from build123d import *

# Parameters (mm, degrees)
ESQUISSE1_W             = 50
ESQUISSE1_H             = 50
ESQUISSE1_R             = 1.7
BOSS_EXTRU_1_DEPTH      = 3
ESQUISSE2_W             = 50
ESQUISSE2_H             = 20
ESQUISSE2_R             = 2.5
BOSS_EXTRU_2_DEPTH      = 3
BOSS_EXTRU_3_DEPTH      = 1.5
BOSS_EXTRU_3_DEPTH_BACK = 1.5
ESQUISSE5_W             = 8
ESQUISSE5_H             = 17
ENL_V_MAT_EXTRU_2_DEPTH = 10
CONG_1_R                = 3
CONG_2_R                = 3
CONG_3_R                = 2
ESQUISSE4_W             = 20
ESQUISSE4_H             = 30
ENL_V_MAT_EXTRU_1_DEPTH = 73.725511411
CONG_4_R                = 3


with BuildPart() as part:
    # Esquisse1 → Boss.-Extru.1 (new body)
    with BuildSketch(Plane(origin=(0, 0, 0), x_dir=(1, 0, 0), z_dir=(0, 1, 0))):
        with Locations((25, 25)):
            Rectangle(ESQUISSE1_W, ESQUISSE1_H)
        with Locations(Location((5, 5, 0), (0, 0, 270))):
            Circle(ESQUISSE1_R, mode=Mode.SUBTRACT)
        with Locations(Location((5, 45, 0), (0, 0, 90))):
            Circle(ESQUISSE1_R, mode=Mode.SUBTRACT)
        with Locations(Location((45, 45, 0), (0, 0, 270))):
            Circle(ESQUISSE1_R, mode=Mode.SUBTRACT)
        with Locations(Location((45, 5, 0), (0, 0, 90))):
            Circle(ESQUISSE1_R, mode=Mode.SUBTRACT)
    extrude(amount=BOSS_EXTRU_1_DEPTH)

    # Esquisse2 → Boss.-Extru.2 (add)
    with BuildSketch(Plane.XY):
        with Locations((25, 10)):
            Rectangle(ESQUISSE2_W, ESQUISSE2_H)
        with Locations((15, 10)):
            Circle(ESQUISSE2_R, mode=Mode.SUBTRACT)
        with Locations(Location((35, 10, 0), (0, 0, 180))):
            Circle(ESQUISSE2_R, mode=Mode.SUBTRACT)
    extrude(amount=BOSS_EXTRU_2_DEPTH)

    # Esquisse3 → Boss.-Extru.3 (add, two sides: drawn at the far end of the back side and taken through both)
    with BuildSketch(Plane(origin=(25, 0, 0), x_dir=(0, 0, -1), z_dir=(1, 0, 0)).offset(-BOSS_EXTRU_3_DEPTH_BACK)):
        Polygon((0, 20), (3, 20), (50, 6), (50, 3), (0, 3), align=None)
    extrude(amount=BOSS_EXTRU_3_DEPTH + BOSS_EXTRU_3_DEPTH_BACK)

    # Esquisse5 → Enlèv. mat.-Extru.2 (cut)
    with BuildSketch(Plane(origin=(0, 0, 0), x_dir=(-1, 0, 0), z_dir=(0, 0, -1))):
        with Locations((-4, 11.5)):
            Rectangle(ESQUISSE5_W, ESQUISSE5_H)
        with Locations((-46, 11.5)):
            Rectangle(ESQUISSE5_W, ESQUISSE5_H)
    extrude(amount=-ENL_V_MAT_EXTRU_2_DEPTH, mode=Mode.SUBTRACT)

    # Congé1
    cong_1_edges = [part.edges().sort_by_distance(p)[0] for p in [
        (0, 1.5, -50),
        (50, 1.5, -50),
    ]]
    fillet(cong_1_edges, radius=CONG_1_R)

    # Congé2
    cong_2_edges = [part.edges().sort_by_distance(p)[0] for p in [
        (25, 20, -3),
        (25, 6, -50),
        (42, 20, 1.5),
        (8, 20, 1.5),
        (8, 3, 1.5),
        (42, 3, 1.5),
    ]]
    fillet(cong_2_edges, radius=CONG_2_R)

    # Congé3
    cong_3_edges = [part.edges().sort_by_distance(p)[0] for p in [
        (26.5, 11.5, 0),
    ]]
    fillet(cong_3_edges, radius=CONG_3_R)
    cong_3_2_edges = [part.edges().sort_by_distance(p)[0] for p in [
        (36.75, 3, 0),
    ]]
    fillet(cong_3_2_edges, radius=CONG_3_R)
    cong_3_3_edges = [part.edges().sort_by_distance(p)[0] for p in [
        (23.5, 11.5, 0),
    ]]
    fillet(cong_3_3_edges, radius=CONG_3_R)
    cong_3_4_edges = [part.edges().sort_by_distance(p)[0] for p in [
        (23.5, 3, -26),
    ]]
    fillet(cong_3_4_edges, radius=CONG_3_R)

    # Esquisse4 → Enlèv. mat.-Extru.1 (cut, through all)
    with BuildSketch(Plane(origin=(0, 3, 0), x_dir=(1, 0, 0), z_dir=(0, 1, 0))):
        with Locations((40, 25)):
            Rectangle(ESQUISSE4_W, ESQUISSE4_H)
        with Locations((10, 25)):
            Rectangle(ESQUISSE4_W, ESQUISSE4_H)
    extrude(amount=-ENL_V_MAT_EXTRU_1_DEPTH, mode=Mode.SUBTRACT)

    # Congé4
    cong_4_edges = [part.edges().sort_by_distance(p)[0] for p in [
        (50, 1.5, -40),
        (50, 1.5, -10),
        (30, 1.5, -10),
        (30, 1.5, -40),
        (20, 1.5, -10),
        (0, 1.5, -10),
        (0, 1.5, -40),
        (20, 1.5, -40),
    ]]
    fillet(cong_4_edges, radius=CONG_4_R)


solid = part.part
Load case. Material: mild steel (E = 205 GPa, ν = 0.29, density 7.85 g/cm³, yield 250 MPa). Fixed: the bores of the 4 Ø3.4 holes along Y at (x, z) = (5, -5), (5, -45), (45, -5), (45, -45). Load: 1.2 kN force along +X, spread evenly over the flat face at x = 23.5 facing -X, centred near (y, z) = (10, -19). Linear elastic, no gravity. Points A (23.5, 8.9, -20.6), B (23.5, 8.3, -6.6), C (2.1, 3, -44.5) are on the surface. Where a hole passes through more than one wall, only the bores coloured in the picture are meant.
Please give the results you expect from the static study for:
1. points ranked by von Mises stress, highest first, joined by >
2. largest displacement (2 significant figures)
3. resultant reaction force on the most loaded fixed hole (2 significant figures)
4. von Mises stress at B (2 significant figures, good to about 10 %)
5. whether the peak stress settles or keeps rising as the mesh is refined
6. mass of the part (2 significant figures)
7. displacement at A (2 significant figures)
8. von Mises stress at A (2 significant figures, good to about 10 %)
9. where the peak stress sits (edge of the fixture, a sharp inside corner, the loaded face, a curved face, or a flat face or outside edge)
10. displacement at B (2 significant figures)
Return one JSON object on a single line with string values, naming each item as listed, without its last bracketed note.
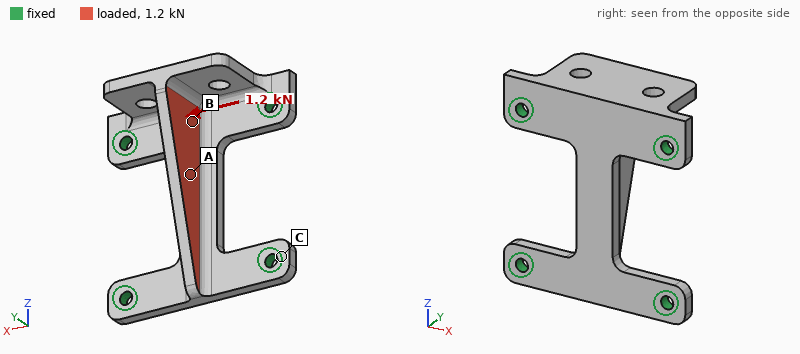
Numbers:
{"points ranked by von Mises stress, highest first, joined by >": "B > A > C", "largest displacement": "36 µm", "resultant reaction force on the most loaded fixed hole": "470 N", "von Mises stress at B": "58 MPa", "whether the peak stress settles or keeps rising as the mesh is refined": "keeps rising", "mass of the part": "59 g", "displacement at A": "21 µm", "von Mises stress at A": "33 MPa", "where the peak stress sits": "edge of the fixture", "displacement at B": "8.1 µm"}
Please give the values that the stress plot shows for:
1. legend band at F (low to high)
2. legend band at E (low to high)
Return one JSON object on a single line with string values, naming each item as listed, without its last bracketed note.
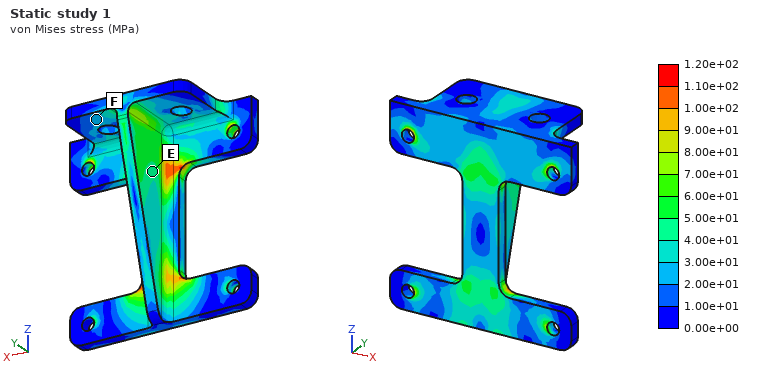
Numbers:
{"legend band at F": "2.00e+01 to 3.00e+01 MPa", "legend band at E": "4.00e+01 to 5.00e+01 MPa"}
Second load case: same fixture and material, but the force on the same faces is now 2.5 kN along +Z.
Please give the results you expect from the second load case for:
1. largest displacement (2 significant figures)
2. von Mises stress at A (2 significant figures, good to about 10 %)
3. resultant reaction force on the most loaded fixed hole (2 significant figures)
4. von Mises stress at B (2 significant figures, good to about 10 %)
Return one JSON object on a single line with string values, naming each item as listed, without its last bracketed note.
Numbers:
{"largest displacement": "31 µm", "von Mises stress at A": "32 MPa", "resultant reaction force on the most loaded fixed hole": "810 N", "von Mises stress at B": "28 MPa"}
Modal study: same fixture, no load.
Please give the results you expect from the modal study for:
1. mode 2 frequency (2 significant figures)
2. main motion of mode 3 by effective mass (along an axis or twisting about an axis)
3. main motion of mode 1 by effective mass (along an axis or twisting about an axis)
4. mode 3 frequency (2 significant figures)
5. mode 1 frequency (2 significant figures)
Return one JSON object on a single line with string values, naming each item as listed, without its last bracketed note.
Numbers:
{"mode 2 frequency": "8700 Hz", "main motion of mode 3 by effective mass": "along X", "main motion of mode 1 by effective mass": "along Y", "mode 3 frequency": "10 kHz", "mode 1 frequency": "6400 Hz"}
